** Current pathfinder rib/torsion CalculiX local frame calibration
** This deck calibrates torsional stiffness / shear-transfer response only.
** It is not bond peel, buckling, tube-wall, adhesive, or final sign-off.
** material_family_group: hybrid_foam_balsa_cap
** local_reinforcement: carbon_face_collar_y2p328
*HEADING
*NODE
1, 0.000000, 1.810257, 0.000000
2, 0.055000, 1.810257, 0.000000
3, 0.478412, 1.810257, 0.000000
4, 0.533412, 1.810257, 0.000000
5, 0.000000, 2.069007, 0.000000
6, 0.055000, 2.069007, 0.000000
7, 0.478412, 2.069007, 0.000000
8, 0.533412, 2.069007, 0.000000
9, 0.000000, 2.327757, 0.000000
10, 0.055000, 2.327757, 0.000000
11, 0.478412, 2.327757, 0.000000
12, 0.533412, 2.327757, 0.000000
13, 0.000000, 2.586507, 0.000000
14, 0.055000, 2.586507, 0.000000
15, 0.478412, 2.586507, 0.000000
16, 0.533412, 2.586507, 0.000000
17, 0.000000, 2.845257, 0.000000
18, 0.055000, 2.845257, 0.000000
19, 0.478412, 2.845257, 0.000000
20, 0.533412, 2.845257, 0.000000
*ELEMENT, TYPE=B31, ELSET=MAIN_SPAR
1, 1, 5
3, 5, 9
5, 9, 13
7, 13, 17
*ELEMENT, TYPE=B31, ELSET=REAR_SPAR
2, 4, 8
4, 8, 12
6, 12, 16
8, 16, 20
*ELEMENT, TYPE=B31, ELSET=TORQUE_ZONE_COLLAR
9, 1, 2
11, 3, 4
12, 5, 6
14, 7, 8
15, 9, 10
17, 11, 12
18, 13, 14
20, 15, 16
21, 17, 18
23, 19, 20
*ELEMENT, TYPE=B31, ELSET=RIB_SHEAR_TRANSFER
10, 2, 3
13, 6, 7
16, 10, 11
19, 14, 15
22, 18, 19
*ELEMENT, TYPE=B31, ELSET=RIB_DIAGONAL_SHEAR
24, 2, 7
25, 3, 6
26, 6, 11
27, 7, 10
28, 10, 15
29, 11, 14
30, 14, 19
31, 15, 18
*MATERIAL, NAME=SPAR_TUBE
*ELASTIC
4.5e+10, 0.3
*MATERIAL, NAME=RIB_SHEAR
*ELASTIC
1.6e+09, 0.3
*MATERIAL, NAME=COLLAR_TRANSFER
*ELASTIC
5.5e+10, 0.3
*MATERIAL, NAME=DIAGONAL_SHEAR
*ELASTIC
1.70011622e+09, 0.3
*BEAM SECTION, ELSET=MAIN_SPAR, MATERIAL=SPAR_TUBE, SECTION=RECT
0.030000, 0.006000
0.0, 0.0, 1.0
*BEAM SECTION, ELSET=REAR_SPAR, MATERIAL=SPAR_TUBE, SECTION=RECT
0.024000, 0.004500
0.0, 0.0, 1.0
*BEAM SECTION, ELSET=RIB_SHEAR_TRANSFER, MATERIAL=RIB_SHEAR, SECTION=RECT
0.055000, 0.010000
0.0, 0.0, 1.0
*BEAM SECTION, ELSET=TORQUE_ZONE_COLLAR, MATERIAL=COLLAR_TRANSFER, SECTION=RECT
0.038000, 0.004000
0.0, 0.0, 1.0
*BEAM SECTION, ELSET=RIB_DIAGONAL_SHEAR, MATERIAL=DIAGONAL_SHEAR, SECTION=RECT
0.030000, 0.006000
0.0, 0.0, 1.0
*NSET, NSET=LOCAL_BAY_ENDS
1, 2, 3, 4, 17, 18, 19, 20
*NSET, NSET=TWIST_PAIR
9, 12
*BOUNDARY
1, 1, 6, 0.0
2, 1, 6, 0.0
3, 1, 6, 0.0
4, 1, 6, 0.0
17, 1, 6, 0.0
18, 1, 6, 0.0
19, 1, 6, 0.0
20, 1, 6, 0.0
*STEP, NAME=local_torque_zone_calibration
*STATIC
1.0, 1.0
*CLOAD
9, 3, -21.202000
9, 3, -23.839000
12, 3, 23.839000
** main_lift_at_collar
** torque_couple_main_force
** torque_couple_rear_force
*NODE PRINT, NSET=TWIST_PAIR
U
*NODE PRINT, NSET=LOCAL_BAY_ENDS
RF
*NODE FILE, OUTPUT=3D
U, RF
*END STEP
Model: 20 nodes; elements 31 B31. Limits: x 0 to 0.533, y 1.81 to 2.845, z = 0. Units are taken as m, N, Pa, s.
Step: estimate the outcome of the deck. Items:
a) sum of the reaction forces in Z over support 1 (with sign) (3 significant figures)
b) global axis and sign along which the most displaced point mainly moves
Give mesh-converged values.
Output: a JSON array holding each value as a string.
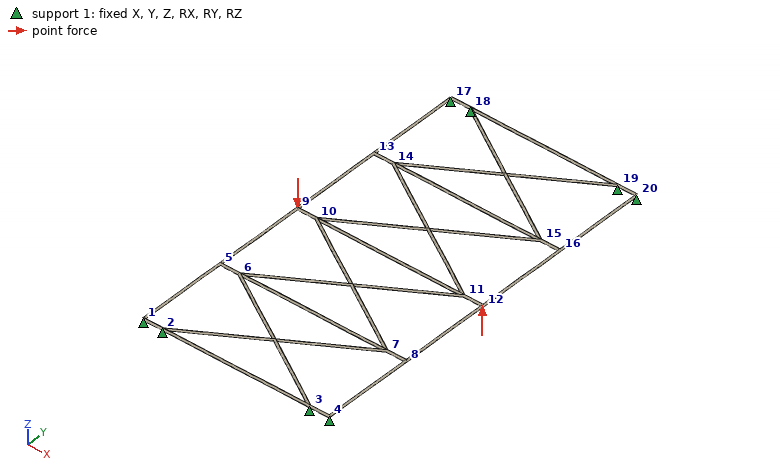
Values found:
["21.2 N", "+Z"]
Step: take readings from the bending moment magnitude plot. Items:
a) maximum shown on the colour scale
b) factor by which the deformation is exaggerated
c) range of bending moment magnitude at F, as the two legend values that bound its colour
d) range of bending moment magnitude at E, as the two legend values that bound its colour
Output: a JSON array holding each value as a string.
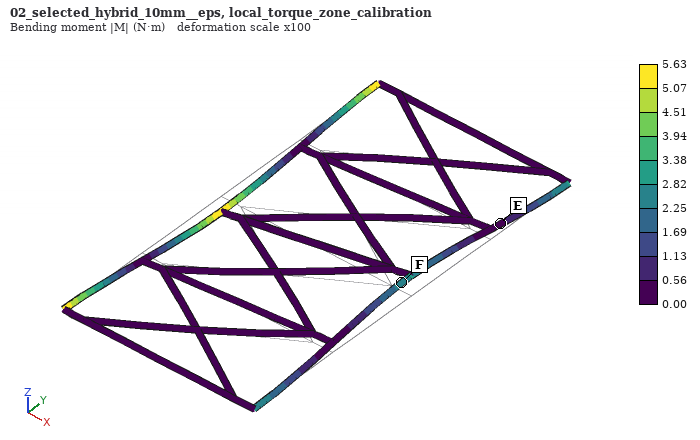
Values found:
["5.63 N·m", "100", "2.25 to 2.82 N·m", "0.00 to 0.56 N·m"]
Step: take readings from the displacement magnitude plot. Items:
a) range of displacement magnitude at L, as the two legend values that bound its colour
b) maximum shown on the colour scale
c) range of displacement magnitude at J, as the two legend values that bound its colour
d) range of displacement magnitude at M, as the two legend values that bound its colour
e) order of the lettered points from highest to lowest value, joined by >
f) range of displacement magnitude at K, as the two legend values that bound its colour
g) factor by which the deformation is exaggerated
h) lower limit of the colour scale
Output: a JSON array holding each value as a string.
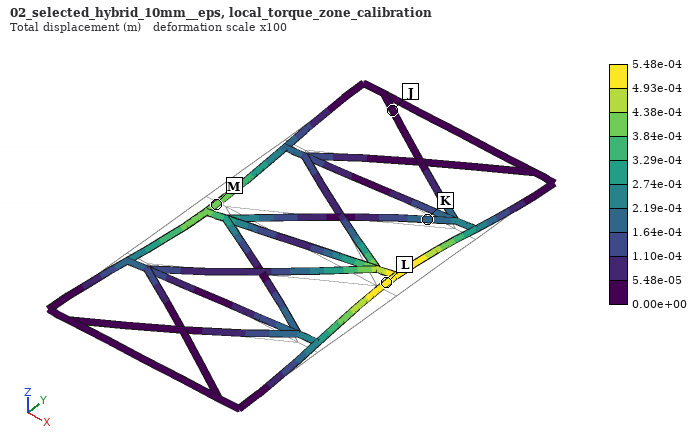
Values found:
["4.93e-04 to 5.48e-04 m", "5.48e-04 m", "0.00e+00 to 5.48e-05 m", "3.84e-04 to 4.38e-04 m", "L > M > K > J", "1.64e-04 to 2.19e-04 m", "100", "0.00e+00 m"]
